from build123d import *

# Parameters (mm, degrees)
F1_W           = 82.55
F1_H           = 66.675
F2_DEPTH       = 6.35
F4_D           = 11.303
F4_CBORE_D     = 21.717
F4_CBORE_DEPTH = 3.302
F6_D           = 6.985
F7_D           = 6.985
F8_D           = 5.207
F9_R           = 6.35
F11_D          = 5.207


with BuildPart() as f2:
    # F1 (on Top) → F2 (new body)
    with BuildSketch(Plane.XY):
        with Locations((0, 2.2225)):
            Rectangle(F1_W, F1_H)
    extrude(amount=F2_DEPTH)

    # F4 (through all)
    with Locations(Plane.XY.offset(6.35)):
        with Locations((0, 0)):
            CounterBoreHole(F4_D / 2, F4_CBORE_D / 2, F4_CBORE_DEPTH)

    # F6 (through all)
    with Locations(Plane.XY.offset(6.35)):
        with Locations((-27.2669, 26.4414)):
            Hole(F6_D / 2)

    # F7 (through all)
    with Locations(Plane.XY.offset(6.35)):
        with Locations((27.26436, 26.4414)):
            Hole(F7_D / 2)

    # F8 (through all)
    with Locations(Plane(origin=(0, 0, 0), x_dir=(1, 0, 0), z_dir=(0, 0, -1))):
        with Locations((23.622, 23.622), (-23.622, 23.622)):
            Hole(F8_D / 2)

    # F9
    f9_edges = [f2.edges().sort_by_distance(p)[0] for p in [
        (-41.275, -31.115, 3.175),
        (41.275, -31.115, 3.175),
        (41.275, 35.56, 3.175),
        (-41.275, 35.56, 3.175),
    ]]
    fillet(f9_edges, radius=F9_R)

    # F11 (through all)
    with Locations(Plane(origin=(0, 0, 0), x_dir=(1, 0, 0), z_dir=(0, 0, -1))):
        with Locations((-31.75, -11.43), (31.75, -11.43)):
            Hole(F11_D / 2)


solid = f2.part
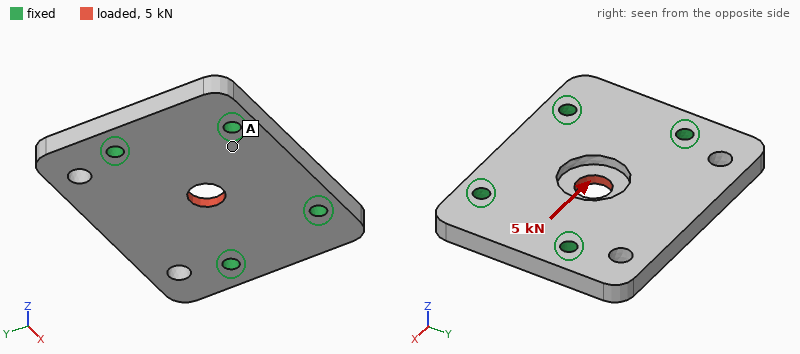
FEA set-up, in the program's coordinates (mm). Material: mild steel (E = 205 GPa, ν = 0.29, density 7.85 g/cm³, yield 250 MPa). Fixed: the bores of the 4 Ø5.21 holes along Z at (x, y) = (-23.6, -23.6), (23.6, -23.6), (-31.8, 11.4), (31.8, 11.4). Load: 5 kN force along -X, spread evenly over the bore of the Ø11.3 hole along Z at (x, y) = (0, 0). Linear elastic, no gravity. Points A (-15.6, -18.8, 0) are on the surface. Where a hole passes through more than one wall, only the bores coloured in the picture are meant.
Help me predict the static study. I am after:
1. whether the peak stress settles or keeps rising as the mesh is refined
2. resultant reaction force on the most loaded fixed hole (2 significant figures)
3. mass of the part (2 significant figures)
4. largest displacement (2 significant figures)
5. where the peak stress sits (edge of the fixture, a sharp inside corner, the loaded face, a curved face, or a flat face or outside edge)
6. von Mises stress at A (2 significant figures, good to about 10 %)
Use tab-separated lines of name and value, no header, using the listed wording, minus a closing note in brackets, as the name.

whether the peak stress settles or keeps rising as the mesh is refined	keeps rising
resultant reaction force on the most loaded fixed hole	1.5 kN
mass of the part	250 g
largest displacement	3.5 µm
where the peak stress sits	a sharp inside corner
von Mises stress at A	12 MPa
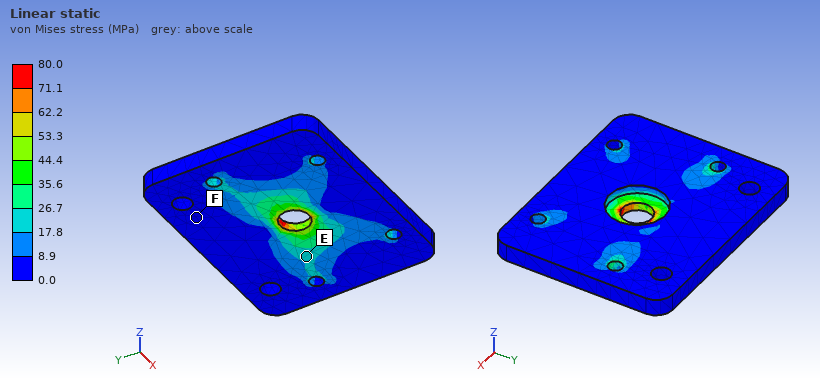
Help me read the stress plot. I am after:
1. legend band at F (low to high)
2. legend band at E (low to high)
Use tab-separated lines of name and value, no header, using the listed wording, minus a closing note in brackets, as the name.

legend band at F	0.0 to 8.9 MPa
legend band at E	17.8 to 26.7 MPa
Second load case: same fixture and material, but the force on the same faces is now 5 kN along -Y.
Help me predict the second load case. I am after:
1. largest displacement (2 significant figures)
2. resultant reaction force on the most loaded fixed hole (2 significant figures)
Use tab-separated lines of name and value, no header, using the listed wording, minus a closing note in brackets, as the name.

largest displacement	4.6 µm
resultant reaction force on the most loaded fixed hole	1.6 kN
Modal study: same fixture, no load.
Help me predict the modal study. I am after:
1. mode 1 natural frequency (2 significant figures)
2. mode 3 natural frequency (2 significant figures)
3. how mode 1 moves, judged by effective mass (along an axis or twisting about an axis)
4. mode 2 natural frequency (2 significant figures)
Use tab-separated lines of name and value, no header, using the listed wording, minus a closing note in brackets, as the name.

mode 1 natural frequency	5600 Hz
mode 3 natural frequency	10 kHz
how mode 1 moves, judged by effective mass	along Z
mode 2 natural frequency	10 kHz
